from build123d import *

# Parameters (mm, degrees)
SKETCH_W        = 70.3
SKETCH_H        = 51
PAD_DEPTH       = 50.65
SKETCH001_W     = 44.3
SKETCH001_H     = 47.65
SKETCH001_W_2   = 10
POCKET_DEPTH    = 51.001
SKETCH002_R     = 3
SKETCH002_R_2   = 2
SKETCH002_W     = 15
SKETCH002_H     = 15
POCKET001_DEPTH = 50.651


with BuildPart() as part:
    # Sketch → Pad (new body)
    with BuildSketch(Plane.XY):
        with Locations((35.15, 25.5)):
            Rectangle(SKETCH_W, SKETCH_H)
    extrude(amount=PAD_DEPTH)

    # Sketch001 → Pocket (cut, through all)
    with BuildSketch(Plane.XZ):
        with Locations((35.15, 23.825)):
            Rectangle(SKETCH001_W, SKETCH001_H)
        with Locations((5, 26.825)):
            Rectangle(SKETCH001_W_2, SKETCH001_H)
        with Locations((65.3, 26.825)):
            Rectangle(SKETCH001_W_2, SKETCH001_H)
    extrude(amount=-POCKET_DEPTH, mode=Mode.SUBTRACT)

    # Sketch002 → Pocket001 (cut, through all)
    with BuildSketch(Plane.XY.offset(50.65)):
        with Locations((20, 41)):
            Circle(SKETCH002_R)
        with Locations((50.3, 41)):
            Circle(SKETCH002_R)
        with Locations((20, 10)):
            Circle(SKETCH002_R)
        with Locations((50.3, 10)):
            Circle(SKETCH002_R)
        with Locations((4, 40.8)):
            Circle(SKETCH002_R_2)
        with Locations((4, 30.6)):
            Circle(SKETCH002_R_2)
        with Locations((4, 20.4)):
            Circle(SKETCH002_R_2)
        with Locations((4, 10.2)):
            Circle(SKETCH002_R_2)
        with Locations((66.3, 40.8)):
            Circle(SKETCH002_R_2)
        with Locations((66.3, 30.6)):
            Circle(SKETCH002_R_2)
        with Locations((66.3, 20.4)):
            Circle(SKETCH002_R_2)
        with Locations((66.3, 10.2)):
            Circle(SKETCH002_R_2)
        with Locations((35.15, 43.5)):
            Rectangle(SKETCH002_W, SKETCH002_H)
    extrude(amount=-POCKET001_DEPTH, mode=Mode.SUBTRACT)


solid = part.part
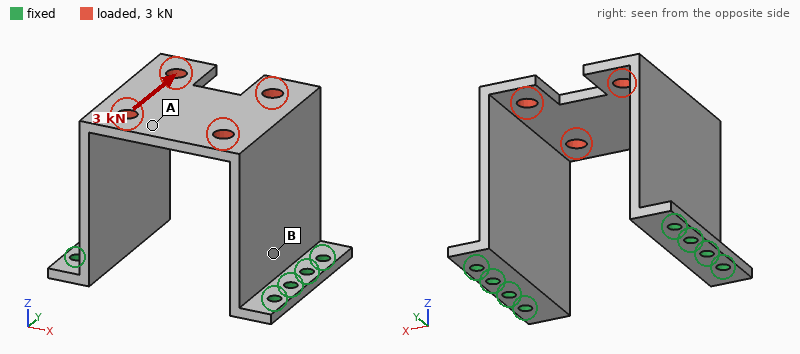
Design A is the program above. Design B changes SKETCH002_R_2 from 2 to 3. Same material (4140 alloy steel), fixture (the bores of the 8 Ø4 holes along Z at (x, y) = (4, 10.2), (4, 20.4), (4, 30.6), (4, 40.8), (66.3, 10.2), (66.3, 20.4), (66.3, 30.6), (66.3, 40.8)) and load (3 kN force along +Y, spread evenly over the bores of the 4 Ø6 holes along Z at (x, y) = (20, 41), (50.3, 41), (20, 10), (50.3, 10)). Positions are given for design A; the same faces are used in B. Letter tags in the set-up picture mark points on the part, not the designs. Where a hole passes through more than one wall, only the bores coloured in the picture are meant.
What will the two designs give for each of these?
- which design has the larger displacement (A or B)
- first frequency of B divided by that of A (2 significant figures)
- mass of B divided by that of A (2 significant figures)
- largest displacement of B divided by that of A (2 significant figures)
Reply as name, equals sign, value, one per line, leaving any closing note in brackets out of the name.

which design has the larger displacement = A
first frequency of B divided by that of A = 1.0
mass of B divided by that of A = 0.98
largest displacement of B divided by that of A = 0.71
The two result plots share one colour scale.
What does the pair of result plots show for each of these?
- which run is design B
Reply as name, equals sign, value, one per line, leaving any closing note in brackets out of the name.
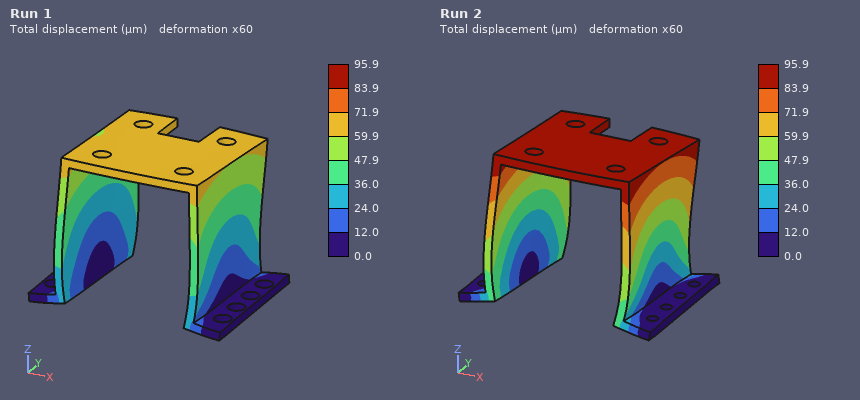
which run is design B = Run 1
